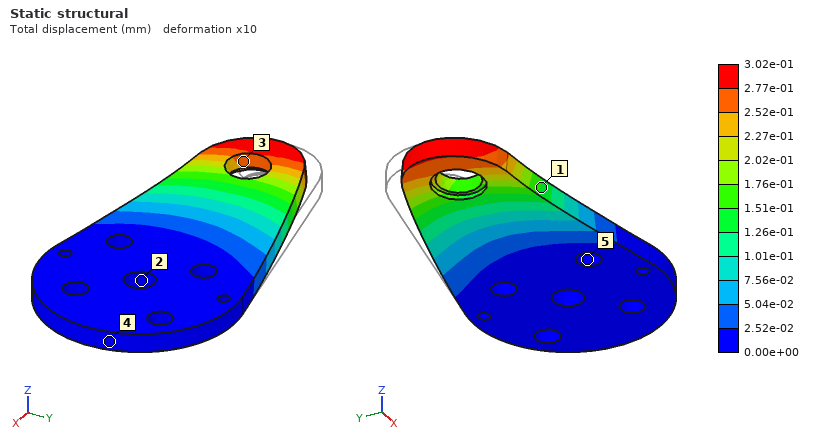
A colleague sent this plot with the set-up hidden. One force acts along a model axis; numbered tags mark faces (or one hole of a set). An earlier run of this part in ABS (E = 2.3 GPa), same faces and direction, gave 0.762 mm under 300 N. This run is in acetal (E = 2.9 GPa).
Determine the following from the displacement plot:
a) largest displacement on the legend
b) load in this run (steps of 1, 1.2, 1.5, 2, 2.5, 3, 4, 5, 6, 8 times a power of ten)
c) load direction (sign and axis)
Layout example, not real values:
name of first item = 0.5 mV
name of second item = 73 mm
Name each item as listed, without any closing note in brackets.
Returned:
largest displacement on the legend = 3.02e-01 mm
load in this run = 150 N
load direction = -Y
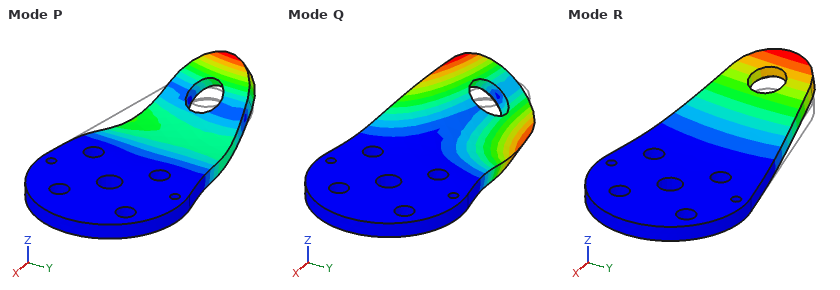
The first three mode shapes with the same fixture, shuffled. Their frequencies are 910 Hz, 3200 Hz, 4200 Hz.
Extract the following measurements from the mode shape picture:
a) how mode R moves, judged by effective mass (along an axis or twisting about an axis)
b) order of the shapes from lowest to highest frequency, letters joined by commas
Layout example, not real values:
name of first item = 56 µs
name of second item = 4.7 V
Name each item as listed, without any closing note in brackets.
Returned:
how mode R moves, judged by effective mass = along Z
order of the shapes from lowest to highest frequency, letters joined by commas = R, Q, P
